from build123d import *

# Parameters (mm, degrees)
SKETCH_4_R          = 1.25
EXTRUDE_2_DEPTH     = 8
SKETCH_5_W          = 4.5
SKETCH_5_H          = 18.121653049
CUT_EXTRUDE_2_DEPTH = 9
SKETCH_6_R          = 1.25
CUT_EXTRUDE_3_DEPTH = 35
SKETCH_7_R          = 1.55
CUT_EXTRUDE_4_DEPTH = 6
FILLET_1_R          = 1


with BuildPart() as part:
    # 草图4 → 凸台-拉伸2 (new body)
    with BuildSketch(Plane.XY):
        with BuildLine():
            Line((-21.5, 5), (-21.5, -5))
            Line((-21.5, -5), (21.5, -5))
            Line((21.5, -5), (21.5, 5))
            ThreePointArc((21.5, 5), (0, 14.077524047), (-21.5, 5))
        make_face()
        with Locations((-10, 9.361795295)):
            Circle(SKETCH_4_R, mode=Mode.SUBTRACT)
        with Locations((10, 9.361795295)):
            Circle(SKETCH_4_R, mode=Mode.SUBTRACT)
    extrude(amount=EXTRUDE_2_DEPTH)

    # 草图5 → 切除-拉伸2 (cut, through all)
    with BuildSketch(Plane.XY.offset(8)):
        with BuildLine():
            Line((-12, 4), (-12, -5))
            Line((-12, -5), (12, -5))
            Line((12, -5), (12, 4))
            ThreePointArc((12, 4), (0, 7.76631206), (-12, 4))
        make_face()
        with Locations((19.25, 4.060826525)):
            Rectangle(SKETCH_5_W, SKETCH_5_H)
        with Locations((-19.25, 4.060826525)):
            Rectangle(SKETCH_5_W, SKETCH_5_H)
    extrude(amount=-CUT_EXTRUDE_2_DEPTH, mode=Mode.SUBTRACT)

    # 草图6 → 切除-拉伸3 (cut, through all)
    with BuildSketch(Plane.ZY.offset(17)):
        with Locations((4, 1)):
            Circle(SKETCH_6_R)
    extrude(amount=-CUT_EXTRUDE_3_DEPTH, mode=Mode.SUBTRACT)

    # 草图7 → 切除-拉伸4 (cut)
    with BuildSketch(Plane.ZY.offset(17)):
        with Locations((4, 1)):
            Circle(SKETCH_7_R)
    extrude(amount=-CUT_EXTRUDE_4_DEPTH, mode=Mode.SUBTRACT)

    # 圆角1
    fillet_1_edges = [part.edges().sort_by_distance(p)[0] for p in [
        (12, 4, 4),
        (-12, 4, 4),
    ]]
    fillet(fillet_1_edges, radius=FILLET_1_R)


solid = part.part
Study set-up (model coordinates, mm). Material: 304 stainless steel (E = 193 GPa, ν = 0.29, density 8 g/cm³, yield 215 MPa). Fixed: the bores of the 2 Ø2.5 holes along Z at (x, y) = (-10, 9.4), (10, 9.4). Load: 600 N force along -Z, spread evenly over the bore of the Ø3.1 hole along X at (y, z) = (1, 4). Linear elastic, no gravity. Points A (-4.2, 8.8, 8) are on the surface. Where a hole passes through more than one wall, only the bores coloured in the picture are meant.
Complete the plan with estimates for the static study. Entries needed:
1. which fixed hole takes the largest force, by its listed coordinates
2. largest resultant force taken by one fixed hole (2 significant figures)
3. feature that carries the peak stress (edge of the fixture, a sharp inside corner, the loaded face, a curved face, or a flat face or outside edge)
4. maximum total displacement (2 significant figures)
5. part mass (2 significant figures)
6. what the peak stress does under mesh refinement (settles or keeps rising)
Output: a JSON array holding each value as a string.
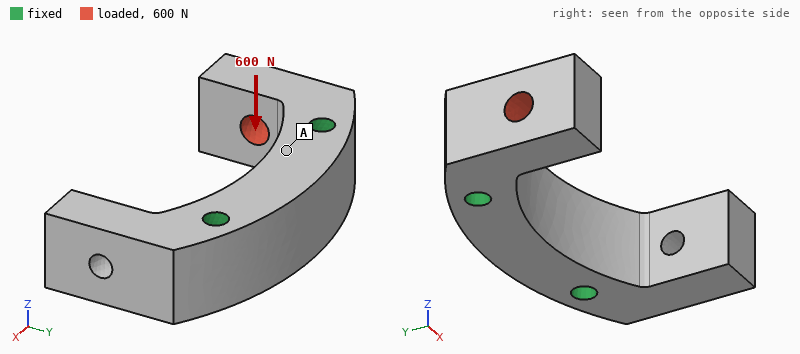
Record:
["(-10, 9.4)", "610 N", "edge of the fixture", "11 µm", "19 g", "keeps rising"]
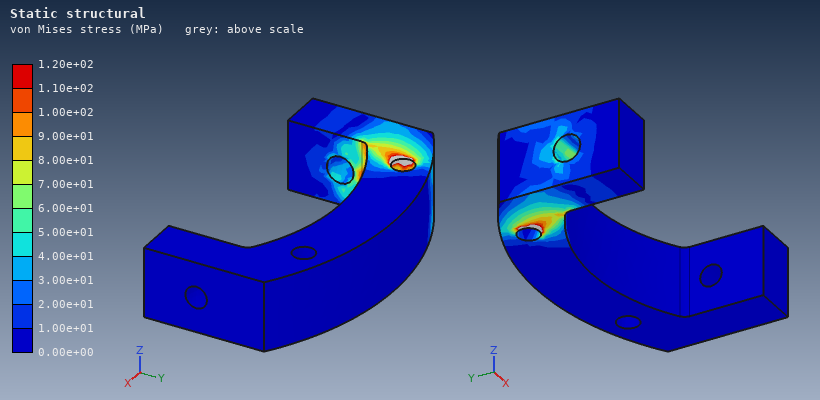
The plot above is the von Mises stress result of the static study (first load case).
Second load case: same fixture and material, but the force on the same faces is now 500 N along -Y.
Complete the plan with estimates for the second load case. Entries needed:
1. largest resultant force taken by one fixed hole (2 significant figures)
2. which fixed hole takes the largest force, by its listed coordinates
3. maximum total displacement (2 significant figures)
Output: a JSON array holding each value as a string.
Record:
["530 N", "(-10, 9.4)", "5.0 µm"]
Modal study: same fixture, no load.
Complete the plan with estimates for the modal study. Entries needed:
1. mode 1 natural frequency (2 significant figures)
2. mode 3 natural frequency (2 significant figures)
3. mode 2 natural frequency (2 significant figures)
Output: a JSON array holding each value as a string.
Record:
["18 kHz", "23 kHz", "18 kHz"]
